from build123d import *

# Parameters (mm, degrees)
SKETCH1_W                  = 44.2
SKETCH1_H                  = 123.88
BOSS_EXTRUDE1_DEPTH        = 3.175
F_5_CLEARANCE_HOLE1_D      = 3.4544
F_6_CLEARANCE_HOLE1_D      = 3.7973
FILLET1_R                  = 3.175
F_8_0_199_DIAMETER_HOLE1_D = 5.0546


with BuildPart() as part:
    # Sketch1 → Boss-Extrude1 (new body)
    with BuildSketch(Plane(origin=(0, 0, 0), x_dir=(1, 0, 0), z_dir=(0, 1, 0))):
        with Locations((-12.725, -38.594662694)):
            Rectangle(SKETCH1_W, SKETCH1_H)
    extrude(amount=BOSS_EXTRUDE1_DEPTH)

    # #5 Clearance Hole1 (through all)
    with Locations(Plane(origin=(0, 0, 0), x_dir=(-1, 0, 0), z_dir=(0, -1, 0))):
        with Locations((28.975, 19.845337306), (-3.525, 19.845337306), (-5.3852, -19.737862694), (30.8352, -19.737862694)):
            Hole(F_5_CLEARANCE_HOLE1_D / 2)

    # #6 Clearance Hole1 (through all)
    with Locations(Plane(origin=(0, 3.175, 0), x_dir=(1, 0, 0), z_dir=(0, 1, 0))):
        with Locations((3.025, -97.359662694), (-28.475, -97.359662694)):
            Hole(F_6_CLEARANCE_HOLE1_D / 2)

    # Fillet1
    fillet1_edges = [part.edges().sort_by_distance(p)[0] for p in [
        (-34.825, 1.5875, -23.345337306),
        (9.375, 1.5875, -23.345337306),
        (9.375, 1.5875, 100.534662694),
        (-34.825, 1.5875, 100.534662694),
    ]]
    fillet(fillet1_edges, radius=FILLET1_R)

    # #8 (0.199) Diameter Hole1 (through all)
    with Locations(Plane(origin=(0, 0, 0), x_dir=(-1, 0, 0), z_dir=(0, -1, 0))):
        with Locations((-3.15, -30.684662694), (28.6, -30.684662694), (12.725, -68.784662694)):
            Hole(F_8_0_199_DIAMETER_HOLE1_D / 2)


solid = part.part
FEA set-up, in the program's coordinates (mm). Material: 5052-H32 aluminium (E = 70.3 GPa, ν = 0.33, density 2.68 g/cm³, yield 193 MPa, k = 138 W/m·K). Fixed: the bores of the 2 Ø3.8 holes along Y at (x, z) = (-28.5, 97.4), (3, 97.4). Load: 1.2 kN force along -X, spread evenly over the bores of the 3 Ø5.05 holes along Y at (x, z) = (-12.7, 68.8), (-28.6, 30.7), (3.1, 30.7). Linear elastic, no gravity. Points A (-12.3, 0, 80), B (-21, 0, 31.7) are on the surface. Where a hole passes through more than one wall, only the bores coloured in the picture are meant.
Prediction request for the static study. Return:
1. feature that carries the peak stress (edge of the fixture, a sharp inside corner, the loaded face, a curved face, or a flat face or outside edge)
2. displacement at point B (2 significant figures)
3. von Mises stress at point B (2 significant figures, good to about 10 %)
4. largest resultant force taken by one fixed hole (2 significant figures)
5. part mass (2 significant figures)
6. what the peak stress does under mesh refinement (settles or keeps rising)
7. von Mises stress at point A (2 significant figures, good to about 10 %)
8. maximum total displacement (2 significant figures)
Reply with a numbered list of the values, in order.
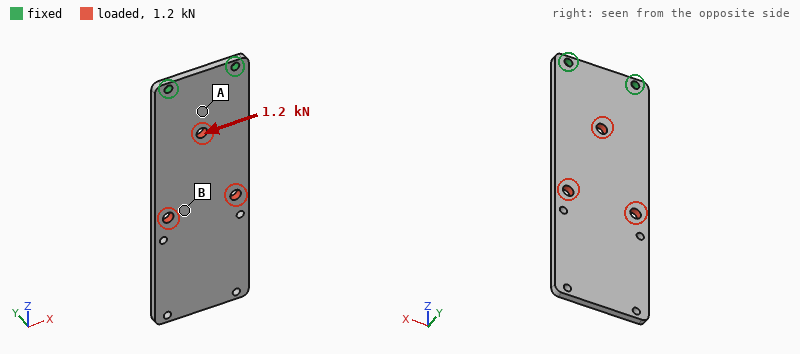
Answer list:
1. edge of the fixture
2. 0.083 mm
3. 10 MPa
4. 2.0 kN
5. 45 g
6. keeps rising
7. 24 MPa
8. 0.16 mm
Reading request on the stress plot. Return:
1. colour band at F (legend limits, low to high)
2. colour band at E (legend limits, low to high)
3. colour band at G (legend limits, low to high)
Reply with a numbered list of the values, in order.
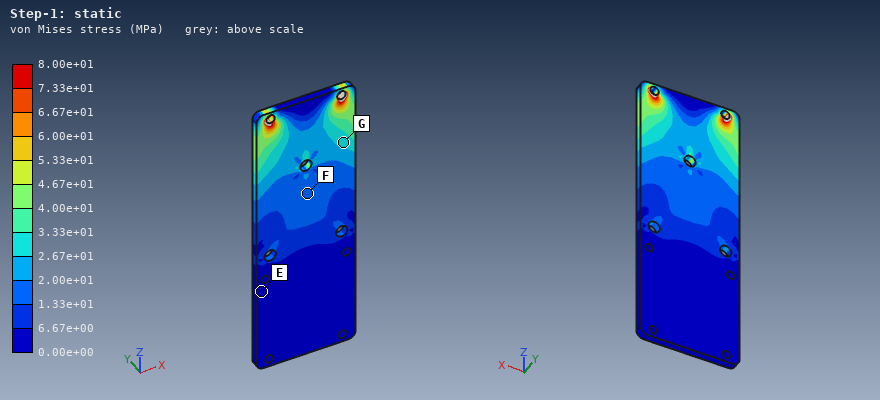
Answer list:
1. 1.33e+01 to 2.00e+01 MPa
2. 0.00e+00 to 6.67e+00 MPa
3. 2.67e+01 to 3.33e+01 MPa
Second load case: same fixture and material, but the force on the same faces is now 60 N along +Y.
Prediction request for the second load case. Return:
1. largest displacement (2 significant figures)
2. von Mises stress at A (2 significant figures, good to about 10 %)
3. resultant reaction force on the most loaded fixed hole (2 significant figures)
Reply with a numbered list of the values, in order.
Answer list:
1. 1.3 mm
2. 27 MPa
3. 30 N
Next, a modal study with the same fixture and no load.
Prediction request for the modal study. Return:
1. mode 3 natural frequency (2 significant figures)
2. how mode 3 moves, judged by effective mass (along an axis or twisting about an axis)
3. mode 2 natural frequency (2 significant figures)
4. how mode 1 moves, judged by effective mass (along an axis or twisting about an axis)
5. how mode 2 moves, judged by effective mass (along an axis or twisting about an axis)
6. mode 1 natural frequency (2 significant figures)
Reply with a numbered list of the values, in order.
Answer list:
1. 1100 Hz
2. along Y
3. 1000 Hz
4. along Y
5. twisting about Z
6. 180 Hz
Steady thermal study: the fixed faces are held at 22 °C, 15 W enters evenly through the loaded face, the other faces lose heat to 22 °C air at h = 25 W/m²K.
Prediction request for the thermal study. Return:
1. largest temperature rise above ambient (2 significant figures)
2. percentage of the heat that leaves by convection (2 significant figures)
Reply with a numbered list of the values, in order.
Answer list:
1. 30 K
2. 38 %
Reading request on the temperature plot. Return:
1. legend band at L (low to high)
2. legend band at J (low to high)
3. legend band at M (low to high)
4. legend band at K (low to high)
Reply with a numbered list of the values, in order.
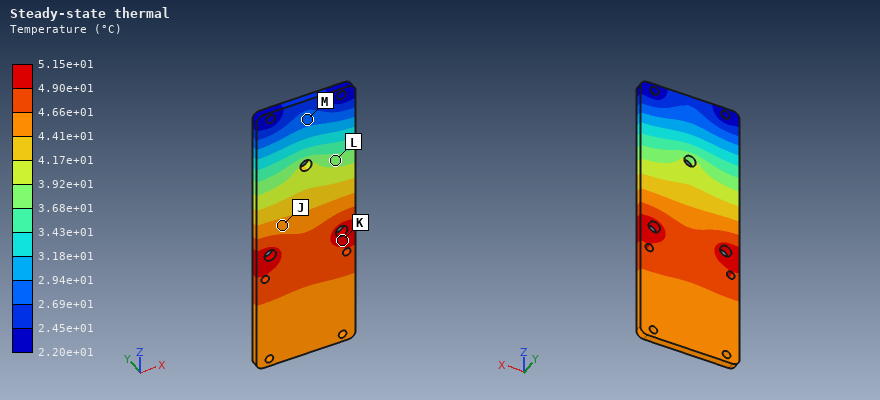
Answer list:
1. 3.68e+01 to 3.92e+01 °C
2. 4.41e+01 to 4.66e+01 °C
3. 2.69e+01 to 2.94e+01 °C
4. 4.90e+01 to 5.15e+01 °C
